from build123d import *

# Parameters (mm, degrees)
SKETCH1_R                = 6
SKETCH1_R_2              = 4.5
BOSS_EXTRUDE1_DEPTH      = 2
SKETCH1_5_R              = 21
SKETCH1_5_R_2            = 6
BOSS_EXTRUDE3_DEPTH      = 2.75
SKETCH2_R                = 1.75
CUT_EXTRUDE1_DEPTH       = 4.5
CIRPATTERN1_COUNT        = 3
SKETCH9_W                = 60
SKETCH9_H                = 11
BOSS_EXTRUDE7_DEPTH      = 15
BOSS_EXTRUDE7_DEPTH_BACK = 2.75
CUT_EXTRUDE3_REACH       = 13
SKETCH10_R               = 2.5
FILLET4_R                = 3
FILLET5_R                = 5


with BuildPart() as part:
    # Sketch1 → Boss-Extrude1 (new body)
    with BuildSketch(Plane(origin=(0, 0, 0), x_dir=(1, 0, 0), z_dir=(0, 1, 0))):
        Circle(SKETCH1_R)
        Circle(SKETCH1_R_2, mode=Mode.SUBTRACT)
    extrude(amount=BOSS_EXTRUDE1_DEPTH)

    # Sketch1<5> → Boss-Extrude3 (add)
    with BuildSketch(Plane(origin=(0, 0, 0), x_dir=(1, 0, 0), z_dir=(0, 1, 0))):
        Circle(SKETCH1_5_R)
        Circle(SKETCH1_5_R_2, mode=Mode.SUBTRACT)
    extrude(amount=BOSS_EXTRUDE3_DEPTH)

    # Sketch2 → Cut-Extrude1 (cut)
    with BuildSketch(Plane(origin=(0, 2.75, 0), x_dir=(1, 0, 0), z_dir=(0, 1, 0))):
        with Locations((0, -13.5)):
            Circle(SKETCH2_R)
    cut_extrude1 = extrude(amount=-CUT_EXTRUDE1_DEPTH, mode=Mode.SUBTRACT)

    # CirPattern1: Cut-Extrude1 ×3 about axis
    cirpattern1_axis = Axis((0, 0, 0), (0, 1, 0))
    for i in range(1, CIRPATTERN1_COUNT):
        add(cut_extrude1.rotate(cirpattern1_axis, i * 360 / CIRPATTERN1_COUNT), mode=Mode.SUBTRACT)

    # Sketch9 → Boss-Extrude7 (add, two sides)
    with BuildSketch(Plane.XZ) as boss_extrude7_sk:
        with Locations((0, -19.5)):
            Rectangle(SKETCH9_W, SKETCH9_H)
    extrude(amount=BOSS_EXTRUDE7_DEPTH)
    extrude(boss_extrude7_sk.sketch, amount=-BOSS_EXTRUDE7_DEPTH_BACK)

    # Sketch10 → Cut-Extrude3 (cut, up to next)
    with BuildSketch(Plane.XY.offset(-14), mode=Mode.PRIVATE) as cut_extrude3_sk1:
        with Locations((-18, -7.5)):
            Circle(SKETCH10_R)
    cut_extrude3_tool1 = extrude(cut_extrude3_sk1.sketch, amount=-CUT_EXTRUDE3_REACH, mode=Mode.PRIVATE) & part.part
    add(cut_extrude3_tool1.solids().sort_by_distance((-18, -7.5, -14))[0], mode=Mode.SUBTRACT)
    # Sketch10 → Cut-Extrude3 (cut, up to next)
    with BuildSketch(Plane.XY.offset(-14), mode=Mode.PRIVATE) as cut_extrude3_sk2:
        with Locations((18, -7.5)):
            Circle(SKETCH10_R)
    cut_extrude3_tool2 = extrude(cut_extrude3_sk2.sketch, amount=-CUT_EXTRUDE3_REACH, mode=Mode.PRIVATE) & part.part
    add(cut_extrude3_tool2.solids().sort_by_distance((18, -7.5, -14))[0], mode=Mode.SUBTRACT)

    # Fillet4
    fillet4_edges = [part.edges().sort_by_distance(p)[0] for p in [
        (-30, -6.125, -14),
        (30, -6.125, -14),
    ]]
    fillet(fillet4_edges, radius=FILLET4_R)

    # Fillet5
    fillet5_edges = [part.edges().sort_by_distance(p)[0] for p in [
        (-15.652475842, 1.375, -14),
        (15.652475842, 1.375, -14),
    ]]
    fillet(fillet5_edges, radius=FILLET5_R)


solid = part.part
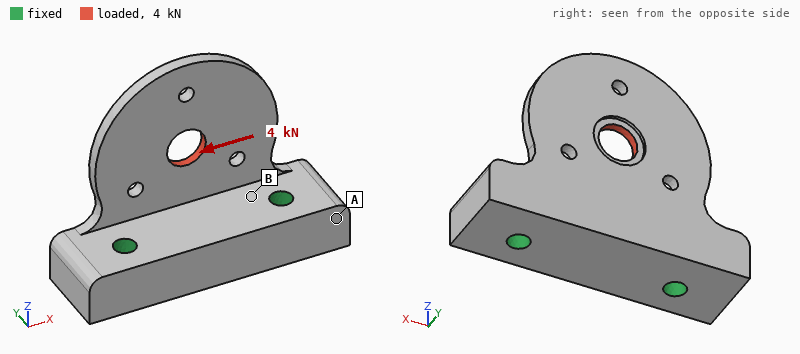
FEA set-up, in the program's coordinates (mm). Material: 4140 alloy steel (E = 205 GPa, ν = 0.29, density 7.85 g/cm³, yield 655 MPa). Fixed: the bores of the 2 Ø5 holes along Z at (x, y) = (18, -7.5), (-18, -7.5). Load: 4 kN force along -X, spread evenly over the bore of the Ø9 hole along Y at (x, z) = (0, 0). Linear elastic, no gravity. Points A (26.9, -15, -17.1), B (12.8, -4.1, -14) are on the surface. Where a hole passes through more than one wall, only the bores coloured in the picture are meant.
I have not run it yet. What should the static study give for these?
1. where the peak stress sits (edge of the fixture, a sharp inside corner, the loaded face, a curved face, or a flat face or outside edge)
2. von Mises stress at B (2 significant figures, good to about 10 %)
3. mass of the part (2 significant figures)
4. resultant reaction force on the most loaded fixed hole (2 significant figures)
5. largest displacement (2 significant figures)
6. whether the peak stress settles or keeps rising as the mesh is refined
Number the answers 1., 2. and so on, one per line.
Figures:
1. a sharp inside corner
2. 37 MPa
3. 110 g
4. 2.9 kN
5. 26 µm
6. keeps rising
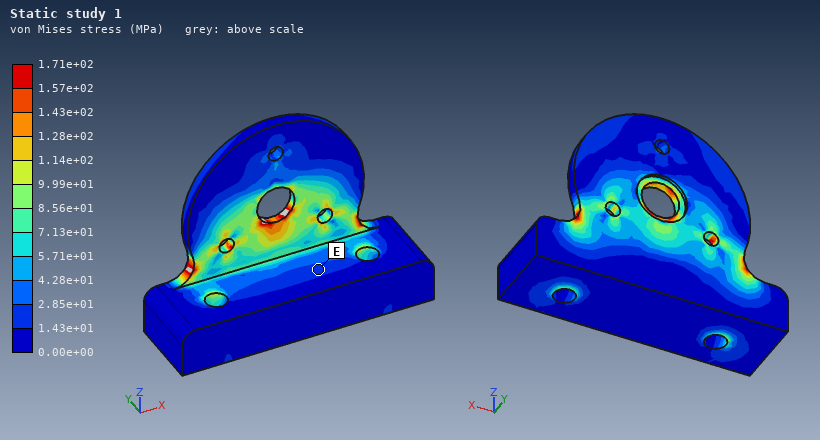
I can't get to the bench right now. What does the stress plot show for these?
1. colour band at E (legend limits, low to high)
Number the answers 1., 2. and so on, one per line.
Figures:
1. 1.43e+01 to 2.85e+01 MPa
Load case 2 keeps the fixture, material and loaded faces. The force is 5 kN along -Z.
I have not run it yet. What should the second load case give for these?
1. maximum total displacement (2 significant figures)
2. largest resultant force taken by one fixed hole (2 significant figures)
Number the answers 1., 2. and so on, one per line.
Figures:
1. 41 µm
2. 2.5 kN
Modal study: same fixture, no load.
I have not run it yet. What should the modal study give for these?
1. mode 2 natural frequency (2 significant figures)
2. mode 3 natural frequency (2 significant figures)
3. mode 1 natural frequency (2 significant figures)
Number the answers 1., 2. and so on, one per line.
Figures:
1. 4900 Hz
2. 10 kHz
3. 2000 Hz
